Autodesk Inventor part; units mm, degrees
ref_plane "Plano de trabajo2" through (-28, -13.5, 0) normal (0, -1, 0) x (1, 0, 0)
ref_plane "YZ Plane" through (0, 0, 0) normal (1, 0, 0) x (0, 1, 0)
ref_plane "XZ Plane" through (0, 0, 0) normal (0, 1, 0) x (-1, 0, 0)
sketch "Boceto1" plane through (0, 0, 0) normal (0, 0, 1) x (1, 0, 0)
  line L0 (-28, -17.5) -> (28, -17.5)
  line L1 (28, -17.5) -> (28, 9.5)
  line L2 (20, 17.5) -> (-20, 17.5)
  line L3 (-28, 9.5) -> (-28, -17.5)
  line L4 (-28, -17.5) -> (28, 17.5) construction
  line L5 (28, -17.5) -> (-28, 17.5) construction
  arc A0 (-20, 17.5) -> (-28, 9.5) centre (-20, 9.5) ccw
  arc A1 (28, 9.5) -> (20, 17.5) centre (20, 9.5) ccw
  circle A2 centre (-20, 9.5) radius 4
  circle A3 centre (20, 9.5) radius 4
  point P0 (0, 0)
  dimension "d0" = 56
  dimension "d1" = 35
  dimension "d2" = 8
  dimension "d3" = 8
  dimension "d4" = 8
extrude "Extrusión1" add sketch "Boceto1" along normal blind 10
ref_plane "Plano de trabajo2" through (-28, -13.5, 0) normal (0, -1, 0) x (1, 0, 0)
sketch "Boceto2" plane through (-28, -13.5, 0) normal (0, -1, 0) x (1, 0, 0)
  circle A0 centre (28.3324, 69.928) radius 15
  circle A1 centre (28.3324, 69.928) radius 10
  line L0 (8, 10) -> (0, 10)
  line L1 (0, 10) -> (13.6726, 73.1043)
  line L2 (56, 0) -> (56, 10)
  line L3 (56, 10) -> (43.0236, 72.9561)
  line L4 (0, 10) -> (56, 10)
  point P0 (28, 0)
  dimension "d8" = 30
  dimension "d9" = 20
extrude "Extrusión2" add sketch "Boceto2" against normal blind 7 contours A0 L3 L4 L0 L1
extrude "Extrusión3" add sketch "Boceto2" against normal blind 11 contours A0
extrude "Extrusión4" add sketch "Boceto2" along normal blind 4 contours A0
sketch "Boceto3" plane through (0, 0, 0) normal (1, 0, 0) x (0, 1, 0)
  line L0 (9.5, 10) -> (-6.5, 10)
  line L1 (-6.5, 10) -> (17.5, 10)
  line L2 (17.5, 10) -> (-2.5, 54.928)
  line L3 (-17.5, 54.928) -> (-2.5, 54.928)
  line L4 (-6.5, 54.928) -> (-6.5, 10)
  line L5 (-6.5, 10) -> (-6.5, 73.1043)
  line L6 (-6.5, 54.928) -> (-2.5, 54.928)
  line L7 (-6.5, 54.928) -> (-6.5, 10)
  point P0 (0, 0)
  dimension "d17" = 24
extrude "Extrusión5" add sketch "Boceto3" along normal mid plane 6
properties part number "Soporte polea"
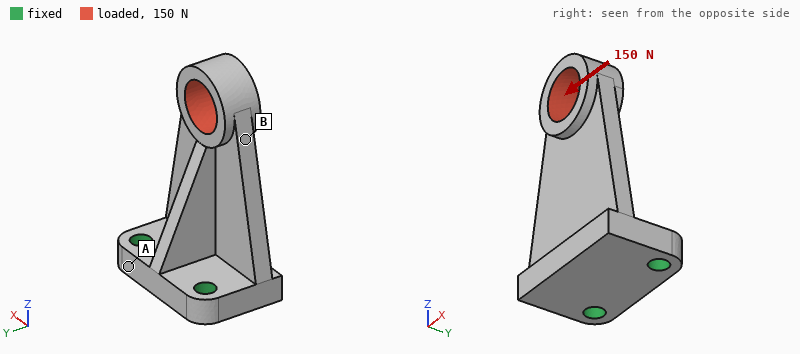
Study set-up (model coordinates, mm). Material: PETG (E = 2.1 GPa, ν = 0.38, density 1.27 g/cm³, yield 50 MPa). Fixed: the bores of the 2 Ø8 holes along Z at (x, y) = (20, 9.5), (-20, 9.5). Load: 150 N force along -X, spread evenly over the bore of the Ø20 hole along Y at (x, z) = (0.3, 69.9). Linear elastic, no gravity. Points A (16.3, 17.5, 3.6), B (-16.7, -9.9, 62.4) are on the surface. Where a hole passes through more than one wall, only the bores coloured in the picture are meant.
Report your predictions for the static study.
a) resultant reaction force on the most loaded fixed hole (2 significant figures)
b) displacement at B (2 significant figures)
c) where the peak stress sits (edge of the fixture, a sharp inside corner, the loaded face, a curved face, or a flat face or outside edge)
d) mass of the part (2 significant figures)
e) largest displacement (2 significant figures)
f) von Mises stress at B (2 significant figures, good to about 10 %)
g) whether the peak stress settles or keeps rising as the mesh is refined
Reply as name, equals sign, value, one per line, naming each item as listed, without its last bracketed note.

resultant reaction force on the most loaded fixed hole = 260 N
displacement at B = 0.33 mm
where the peak stress sits = edge of the fixture
mass of the part = 55 g
largest displacement = 0.50 mm
von Mises stress at B = 2.9 MPa
whether the peak stress settles or keeps rising as the mesh is refined = keeps rising
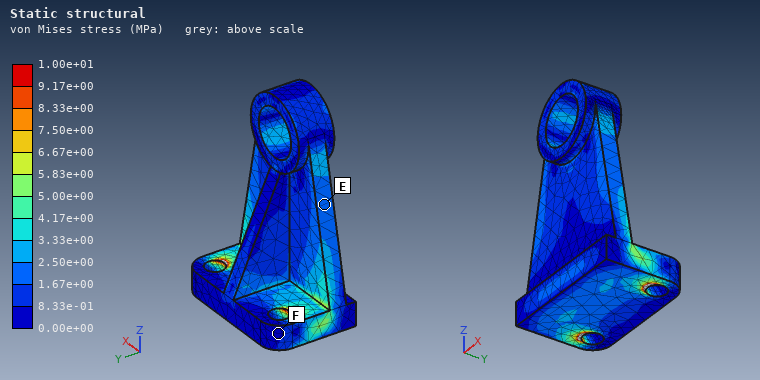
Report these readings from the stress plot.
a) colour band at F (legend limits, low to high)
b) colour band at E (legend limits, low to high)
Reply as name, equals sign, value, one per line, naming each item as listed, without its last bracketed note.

colour band at F = 0.00e+00 to 8.33e-01 MPa
colour band at E = 1.67e+00 to 2.50e+00 MPa
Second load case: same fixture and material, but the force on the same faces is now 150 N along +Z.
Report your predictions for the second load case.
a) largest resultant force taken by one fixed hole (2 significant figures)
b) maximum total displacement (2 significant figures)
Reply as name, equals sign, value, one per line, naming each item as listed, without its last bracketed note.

largest resultant force taken by one fixed hole = 76 N
maximum total displacement = 0.22 mm
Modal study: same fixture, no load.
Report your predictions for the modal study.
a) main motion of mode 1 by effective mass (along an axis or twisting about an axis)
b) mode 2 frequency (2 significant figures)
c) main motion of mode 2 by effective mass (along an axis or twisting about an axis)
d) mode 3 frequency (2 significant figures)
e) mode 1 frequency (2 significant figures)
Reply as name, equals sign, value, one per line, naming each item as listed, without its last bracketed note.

main motion of mode 1 by effective mass = along Y
mode 2 frequency = 880 Hz
main motion of mode 2 by effective mass = along X
mode 3 frequency = 1300 Hz
mode 1 frequency = 500 Hz
